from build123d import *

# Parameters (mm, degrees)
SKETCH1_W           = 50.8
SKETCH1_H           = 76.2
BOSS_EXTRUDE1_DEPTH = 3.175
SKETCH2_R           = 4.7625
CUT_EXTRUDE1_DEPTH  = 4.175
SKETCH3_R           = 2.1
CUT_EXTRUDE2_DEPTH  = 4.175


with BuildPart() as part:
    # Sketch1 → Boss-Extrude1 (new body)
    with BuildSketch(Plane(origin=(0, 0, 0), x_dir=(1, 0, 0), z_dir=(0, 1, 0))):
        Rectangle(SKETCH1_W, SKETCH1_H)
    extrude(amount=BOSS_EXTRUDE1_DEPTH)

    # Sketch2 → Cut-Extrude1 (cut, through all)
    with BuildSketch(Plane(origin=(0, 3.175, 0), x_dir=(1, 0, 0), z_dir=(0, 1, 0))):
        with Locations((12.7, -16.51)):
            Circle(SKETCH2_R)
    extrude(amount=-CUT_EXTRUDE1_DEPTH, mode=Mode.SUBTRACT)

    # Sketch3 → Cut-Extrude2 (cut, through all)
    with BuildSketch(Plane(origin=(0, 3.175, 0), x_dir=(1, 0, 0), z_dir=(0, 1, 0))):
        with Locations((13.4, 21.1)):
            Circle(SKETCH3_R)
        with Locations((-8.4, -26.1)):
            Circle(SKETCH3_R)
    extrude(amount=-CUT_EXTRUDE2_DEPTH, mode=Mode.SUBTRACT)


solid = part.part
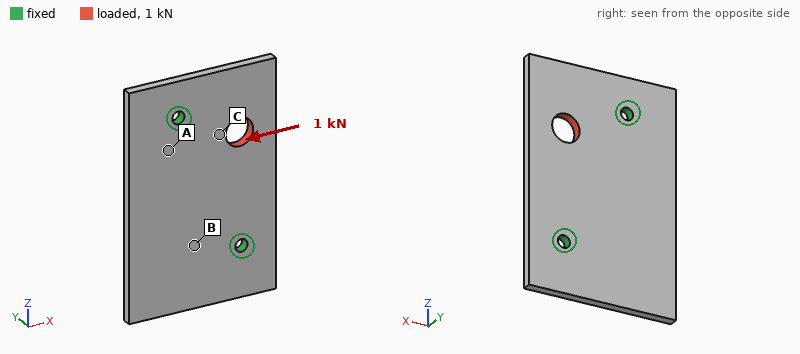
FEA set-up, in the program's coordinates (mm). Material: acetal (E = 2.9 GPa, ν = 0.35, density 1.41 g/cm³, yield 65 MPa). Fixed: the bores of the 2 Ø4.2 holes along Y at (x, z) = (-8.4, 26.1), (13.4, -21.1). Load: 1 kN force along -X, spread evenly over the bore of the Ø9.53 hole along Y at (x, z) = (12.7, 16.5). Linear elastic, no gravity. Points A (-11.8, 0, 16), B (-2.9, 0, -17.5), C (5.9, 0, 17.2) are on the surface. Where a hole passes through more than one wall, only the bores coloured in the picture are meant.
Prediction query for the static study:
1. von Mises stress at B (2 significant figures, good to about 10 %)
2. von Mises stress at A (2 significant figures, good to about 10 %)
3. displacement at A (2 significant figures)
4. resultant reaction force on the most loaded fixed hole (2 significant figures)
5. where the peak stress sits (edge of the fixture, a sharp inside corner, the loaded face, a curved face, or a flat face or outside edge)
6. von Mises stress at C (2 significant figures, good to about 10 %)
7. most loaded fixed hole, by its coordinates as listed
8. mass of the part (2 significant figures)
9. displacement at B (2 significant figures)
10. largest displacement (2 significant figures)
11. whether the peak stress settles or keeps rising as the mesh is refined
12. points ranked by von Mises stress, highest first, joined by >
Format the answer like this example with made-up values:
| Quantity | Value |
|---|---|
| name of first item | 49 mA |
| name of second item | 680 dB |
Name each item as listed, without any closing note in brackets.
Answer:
| Quantity | Value |
|---|---|
| von Mises stress at B | 3.1 MPa |
| von Mises stress at A | 7.0 MPa |
| displacement at A | 0.049 mm |
| resultant reaction force on the most loaded fixed hole | 780 N |
| where the peak stress sits | edge of the fixture |
| von Mises stress at C | 12 MPa |
| most loaded fixed hole, by its coordinates as listed | (-8.4, 26.1) |
| mass of the part | 17 g |
| displacement at B | 0.033 mm |
| largest displacement | 0.16 mm |
| whether the peak stress settles or keeps rising as the mesh is refined | keeps rising |
| points ranked by von Mises stress, highest first, joined by > | C > A > B |
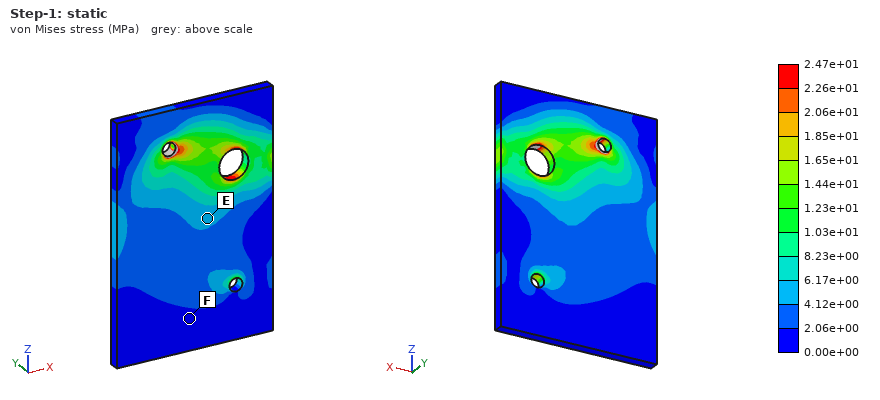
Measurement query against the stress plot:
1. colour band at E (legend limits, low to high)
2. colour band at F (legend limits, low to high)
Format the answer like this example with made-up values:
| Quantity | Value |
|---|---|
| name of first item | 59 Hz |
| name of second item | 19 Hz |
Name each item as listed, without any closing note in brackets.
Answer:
| Quantity | Value |
|---|---|
| colour band at E | 4.12e+00 to 6.17e+00 MPa |
| colour band at F | 0.00e+00 to 2.06e+00 MPa |
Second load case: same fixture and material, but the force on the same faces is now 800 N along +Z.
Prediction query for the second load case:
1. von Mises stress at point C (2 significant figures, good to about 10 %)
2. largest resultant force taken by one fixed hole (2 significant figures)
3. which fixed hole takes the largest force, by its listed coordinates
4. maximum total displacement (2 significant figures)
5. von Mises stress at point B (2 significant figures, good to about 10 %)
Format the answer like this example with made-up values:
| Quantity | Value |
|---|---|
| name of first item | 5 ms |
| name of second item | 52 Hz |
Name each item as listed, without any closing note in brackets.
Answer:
| Quantity | Value |
|---|---|
| von Mises stress at point C | 10 MPa |
| largest resultant force taken by one fixed hole | 460 N |
| which fixed hole takes the largest force, by its listed coordinates | (13.4, -21.1) |
| maximum total displacement | 0.14 mm |
| von Mises stress at point B | 2.1 MPa |
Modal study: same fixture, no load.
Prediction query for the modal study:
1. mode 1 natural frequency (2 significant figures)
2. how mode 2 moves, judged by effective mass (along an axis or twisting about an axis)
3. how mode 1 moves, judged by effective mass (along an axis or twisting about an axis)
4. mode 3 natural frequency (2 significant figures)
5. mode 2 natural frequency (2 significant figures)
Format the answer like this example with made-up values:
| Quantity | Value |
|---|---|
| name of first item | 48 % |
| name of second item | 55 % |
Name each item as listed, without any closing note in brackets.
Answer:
| Quantity | Value |
|---|---|
| mode 1 natural frequency | 570 Hz |
| how mode 2 moves, judged by effective mass | along Y |
| how mode 1 moves, judged by effective mass | along Y |
| mode 3 natural frequency | 1300 Hz |
| mode 2 natural frequency | 830 Hz |
